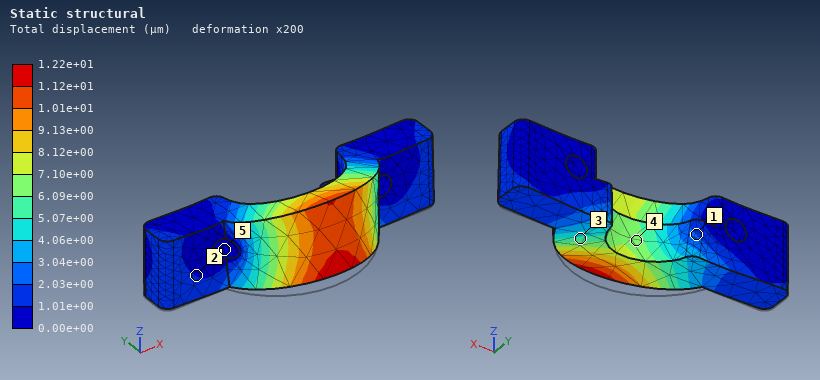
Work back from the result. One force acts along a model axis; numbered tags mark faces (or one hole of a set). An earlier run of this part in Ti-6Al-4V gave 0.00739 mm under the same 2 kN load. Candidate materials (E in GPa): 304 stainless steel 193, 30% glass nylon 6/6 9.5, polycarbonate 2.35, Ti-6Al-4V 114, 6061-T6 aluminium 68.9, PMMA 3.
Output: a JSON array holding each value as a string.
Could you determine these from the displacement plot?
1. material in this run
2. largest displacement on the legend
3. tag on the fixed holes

["6061-T6 aluminium", "1.22e+01 µm", "5"]
